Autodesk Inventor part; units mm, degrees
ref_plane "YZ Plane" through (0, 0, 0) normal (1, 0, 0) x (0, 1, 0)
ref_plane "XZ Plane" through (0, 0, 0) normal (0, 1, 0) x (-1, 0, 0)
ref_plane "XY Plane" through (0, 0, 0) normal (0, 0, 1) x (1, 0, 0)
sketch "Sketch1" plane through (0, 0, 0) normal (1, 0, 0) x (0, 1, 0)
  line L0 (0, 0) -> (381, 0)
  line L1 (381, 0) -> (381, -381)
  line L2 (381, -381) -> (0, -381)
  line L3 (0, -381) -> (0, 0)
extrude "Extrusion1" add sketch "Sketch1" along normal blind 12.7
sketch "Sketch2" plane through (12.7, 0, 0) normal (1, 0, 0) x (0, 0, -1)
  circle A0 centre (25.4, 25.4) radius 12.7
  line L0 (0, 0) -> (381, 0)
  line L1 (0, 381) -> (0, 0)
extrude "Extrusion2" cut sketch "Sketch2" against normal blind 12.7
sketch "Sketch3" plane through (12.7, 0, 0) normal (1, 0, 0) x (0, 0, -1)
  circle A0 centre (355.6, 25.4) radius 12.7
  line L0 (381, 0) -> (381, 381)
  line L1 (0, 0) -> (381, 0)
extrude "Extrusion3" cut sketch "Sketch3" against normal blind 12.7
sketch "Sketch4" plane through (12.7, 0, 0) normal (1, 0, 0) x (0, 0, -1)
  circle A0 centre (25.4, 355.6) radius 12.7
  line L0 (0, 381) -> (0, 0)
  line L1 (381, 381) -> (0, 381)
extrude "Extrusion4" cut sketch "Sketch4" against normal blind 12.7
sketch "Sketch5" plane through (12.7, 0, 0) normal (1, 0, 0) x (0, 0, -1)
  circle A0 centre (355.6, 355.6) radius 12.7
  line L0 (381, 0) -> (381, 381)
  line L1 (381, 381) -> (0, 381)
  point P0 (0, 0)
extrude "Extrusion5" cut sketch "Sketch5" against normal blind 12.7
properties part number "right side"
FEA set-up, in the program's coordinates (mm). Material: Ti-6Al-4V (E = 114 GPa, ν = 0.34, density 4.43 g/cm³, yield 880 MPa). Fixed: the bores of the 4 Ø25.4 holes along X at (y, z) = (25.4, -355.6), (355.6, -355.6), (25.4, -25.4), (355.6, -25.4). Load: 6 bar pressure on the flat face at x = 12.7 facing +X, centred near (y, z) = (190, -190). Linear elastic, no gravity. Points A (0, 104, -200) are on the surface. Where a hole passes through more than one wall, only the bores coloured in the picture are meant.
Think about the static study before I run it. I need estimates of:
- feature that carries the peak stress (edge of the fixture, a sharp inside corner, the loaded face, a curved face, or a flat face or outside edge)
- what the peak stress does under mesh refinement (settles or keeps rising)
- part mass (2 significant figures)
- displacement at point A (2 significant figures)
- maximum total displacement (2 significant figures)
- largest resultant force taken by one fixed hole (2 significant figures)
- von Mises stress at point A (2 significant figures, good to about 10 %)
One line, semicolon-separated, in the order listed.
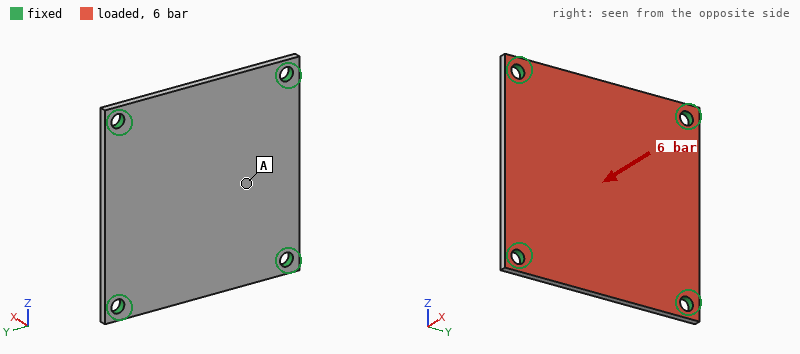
edge of the fixture; keeps rising; 8.1 kg; 1.9 mm; 2.3 mm; 21 kN; 110 MPa
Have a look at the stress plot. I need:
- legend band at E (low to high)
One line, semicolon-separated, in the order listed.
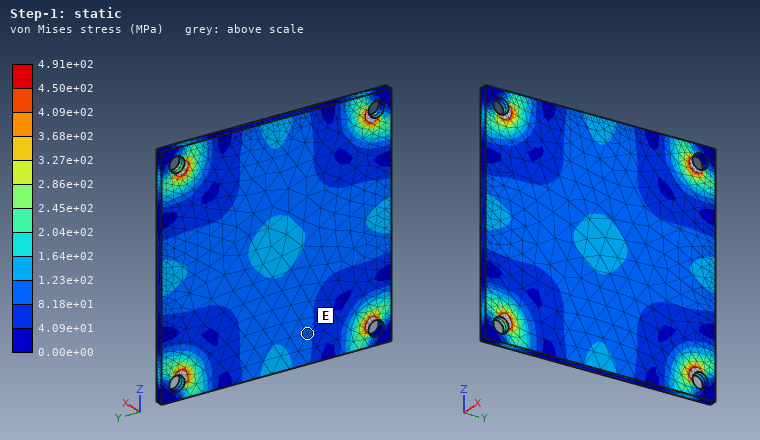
8.18e+01 to 1.23e+02 MPa
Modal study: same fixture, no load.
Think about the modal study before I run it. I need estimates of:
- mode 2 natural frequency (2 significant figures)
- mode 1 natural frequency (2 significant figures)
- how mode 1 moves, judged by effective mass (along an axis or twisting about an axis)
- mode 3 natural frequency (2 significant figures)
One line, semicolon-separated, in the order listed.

720 Hz; 420 Hz; along X; 720 Hz
